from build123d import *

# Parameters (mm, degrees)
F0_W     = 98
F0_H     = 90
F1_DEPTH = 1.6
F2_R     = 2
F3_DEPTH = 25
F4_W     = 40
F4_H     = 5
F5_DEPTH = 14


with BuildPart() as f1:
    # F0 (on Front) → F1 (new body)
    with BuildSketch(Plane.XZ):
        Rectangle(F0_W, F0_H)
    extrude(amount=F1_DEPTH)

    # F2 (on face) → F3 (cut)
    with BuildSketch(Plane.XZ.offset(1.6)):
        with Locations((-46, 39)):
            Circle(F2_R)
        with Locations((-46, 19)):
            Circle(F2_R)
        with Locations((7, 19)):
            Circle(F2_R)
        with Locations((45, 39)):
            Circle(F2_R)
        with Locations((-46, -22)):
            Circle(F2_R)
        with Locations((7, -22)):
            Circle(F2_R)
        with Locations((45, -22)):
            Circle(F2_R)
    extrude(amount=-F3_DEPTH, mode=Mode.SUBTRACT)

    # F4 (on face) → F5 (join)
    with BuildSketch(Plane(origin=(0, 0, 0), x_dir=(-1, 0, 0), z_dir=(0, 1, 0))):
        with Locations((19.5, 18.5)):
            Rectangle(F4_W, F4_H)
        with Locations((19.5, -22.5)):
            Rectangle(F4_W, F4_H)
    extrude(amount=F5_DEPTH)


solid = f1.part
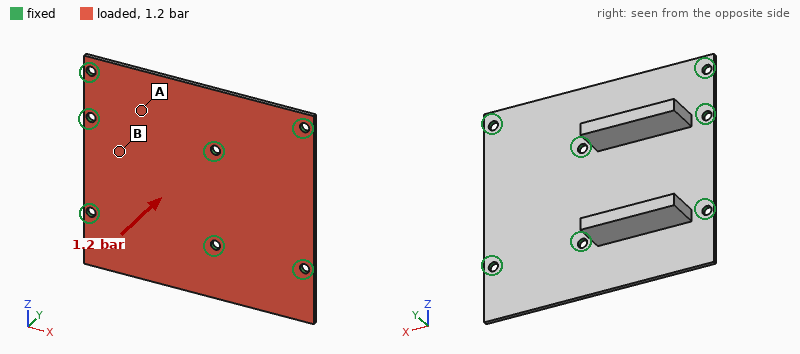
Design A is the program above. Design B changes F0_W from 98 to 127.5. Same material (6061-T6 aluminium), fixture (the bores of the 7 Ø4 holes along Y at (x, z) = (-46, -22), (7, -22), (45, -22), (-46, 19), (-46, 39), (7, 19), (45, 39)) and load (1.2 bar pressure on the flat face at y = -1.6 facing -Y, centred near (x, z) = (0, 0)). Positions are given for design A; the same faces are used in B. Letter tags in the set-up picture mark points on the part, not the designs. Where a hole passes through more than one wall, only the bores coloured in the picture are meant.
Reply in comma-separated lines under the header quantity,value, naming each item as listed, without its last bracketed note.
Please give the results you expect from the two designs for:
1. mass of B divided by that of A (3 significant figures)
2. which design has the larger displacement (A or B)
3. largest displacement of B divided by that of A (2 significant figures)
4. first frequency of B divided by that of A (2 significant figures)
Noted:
quantity,value
mass of B divided by that of A,1.22
which design has the larger displacement,B
largest displacement of B divided by that of A,1.5
first frequency of B divided by that of A,0.94
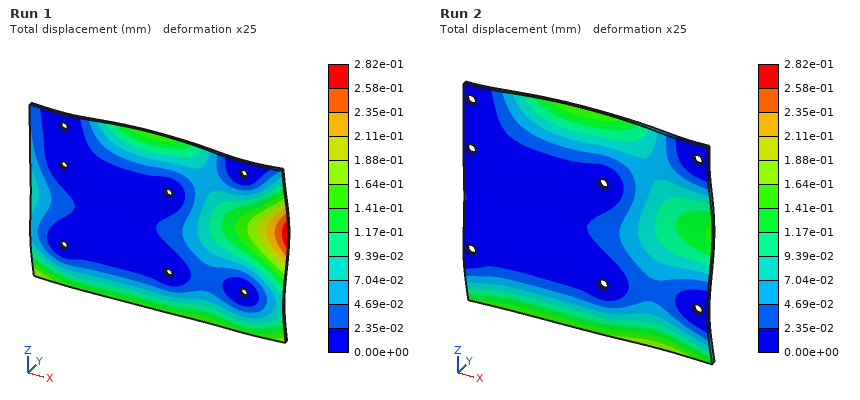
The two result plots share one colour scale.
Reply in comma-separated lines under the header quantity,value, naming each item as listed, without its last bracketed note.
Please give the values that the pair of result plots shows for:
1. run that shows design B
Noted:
quantity,value
run that shows design B,Run 1
